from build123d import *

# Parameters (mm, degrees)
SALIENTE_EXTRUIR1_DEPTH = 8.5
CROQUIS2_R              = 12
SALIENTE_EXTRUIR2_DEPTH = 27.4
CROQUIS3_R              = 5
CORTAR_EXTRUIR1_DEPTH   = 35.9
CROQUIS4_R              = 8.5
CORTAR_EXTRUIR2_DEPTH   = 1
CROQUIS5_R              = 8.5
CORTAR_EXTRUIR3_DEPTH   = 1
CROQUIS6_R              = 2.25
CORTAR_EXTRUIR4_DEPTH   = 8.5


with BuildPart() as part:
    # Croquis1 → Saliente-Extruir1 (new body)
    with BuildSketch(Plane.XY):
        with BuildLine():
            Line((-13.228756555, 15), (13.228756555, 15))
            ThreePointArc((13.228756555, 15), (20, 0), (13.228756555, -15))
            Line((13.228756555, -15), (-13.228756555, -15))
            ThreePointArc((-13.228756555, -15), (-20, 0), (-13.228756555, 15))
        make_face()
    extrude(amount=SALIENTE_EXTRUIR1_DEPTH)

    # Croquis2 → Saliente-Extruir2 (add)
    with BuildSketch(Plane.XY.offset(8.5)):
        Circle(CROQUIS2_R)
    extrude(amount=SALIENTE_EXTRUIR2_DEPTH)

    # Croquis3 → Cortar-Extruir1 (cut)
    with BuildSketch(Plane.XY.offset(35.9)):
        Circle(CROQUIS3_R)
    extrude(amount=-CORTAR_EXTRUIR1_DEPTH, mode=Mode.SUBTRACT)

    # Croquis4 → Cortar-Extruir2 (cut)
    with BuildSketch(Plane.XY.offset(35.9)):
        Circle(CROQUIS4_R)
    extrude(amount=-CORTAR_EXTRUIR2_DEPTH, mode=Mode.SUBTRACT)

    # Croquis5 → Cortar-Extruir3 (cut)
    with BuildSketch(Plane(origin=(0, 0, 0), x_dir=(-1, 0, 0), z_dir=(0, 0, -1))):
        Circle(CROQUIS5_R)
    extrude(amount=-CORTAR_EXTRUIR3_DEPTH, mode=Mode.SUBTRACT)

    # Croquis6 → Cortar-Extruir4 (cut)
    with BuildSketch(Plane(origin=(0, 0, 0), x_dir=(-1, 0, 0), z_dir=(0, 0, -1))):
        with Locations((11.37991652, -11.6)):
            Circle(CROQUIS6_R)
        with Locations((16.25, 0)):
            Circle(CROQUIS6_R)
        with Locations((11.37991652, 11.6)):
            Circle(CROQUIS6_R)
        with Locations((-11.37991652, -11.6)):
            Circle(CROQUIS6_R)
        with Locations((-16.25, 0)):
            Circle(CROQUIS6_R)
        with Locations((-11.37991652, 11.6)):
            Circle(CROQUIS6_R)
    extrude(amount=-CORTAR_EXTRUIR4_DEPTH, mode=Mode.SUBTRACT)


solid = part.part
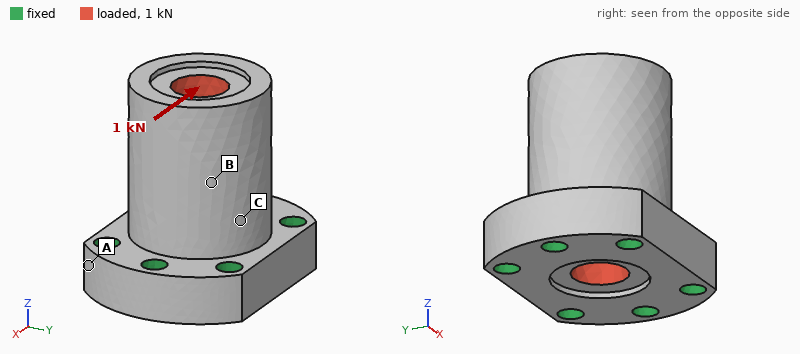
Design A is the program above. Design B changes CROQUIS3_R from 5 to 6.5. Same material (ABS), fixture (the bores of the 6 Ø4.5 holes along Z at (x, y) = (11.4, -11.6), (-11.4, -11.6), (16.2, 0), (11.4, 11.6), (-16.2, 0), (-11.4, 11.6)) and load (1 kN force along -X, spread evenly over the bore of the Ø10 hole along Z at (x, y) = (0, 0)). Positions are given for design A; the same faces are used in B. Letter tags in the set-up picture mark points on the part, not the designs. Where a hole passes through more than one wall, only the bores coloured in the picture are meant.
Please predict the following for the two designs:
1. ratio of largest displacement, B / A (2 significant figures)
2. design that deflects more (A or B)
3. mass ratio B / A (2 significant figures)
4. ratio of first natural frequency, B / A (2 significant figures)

1.1
B
0.90
1.0
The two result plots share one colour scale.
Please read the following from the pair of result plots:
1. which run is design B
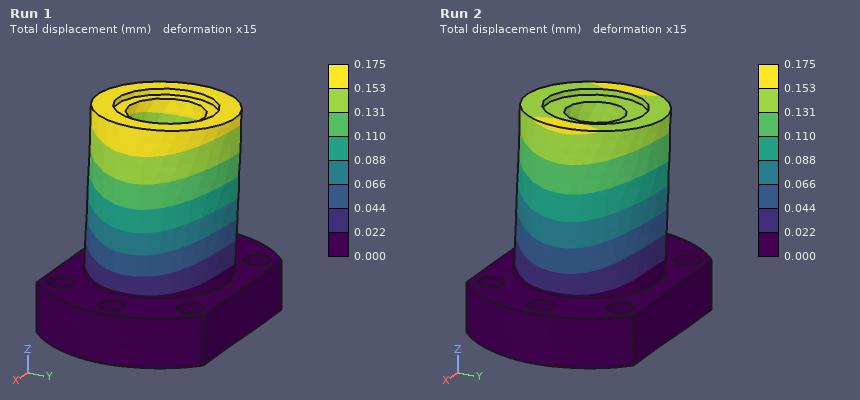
Run 1
